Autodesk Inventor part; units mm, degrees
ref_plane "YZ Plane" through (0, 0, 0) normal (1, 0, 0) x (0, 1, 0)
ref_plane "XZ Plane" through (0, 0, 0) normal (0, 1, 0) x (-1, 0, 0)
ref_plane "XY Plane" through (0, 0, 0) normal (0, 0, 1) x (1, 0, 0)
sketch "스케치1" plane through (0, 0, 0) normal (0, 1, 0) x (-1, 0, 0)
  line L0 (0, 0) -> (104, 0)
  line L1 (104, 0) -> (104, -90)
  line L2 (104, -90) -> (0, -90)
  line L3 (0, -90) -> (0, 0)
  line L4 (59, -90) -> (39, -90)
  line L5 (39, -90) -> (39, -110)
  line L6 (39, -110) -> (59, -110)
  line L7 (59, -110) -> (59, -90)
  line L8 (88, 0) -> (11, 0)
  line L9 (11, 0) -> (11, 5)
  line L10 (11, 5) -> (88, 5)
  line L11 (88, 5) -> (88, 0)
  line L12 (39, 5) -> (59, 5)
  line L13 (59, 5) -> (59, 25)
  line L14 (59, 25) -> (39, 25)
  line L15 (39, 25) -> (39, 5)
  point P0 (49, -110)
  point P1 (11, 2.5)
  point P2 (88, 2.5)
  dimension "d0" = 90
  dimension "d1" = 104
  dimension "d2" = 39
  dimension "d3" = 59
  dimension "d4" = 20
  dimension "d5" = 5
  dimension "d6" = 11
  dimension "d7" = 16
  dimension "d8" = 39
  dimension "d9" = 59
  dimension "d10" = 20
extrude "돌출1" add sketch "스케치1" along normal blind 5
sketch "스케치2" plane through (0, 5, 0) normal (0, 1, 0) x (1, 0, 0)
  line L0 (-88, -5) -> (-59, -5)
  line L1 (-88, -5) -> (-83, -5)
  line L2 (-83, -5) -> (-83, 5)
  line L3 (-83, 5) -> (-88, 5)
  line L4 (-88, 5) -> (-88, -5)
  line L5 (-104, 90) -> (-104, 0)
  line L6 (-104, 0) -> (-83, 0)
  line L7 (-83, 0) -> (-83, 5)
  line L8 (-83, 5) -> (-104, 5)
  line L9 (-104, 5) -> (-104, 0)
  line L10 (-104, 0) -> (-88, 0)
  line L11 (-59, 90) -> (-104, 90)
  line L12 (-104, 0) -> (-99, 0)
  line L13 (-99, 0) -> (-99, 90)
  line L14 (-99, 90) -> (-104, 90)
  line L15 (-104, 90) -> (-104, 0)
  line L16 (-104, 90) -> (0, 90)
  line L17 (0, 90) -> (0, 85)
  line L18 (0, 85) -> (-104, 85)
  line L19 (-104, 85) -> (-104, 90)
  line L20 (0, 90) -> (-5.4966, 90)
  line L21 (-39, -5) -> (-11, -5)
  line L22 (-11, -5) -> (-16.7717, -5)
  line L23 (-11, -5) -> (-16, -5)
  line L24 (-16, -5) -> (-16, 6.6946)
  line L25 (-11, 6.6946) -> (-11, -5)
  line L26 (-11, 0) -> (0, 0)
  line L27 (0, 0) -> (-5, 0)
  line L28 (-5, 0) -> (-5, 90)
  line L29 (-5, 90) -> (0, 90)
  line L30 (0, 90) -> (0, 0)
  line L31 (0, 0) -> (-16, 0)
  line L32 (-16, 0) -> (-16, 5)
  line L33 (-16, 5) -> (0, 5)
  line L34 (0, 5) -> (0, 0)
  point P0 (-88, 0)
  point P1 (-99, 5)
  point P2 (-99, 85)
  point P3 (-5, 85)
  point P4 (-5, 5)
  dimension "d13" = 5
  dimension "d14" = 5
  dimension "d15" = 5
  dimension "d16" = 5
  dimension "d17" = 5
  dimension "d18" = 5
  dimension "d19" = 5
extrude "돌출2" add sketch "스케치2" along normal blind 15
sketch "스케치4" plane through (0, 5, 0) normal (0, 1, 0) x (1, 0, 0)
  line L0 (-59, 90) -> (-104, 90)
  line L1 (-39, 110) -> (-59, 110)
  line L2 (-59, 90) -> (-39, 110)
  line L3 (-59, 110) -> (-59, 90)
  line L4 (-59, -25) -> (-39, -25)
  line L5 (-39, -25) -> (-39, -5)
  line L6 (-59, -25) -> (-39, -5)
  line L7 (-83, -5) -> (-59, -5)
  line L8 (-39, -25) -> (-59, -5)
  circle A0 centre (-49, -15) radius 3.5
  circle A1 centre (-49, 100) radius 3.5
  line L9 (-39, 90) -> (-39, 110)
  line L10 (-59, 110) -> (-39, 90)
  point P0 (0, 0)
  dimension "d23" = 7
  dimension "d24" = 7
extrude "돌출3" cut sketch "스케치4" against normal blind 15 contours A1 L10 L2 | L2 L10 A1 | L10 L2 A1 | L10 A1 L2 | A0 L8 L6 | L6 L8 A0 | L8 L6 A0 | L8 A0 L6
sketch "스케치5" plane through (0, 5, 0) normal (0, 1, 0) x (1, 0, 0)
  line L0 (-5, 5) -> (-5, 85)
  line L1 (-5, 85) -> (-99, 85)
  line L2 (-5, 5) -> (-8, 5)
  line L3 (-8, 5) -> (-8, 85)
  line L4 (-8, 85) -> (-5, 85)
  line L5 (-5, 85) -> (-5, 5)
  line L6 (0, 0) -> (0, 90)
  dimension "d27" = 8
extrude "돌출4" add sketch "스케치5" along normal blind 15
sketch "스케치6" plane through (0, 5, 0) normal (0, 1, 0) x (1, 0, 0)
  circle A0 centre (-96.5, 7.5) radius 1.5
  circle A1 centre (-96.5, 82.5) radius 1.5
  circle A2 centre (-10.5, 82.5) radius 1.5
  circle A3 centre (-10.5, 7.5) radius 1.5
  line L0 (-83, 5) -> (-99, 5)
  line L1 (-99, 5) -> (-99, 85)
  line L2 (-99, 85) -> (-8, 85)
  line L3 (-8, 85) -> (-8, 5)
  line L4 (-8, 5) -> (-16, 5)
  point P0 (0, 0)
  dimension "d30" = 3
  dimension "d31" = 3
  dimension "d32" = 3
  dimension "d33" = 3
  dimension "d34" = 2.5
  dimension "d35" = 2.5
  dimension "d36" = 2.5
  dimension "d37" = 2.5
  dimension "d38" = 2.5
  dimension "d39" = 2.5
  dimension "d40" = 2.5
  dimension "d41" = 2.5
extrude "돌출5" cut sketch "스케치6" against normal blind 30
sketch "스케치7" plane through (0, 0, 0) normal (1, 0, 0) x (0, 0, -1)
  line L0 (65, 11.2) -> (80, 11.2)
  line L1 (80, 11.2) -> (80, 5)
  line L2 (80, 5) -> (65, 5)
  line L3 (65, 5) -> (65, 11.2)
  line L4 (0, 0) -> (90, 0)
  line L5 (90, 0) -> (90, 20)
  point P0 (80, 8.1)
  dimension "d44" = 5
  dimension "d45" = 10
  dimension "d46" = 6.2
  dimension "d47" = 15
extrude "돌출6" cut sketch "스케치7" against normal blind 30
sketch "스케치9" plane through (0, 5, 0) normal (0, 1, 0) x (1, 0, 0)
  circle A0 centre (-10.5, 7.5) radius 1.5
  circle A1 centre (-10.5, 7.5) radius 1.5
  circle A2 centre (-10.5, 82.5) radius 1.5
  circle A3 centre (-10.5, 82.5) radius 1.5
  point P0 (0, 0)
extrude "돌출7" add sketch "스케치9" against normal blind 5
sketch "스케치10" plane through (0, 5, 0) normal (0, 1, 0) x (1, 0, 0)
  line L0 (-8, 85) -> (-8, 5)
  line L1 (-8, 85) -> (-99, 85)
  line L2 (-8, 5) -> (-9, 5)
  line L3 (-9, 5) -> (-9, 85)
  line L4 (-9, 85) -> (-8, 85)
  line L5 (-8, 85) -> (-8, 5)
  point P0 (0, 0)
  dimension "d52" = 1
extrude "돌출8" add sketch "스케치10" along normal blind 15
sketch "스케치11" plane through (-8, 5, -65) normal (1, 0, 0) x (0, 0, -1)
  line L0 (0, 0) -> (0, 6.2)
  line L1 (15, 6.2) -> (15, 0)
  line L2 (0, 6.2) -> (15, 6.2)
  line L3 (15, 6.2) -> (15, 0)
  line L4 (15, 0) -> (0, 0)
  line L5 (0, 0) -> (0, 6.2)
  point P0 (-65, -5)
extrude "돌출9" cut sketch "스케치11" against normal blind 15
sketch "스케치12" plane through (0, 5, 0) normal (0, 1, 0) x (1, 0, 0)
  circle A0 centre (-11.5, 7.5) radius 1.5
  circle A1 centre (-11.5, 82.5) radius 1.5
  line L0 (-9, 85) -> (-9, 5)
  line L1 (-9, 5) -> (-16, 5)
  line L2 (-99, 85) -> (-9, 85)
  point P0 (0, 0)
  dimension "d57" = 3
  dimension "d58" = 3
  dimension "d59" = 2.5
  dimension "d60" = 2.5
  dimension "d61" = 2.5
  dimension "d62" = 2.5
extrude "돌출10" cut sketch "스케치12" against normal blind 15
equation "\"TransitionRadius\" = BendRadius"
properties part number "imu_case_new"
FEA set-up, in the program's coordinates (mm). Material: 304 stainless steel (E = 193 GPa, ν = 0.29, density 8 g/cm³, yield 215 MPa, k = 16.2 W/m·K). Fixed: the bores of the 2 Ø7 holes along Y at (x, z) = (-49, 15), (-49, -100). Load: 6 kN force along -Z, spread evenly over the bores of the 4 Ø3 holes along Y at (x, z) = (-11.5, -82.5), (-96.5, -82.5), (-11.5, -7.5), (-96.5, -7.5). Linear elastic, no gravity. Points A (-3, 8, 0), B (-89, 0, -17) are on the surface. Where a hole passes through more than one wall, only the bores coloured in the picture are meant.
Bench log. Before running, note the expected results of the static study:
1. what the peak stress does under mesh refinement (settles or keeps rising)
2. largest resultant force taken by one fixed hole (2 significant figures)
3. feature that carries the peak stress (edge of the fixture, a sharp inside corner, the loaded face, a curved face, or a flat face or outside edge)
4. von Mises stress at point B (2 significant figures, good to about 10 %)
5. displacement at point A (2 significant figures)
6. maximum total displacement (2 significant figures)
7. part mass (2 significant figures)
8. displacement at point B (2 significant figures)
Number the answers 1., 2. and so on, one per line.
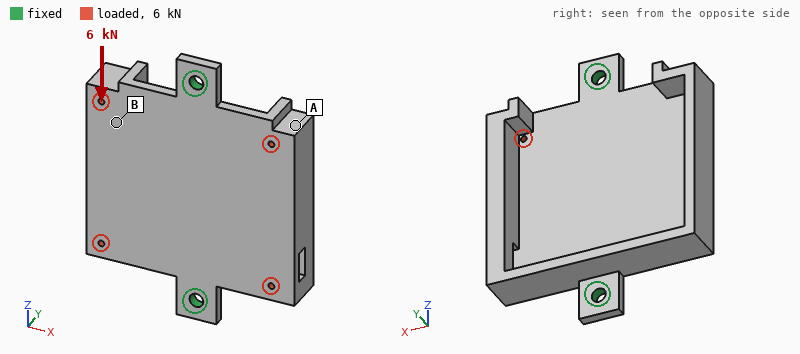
1. keeps rising
2. 3.1 kN
3. edge of the fixture
4. 15 MPa
5. 6.5 µm
6. 12 µm
7. 640 g
8. 7.7 µm
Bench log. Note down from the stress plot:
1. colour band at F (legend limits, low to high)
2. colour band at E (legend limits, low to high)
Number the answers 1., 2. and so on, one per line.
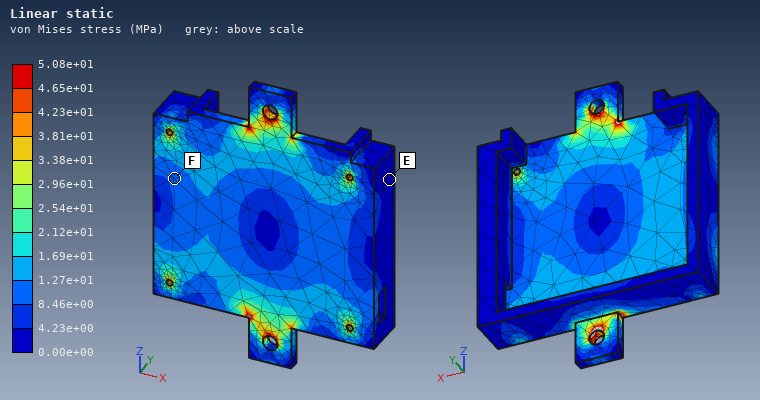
1. 8.46e+00 to 1.27e+01 MPa
2. 0.00e+00 to 4.23e+00 MPa
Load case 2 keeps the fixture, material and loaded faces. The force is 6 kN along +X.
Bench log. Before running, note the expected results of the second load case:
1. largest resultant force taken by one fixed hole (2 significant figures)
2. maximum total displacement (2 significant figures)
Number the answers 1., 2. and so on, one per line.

1. 3.1 kN
2. 13 µm
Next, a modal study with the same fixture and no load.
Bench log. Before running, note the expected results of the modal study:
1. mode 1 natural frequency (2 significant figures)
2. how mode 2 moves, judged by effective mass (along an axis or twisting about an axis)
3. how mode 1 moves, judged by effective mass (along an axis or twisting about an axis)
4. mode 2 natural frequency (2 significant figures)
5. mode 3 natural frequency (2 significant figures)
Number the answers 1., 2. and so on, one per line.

1. 590 Hz
2. along Y
3. twisting about Z
4. 1100 Hz
5. 1800 Hz
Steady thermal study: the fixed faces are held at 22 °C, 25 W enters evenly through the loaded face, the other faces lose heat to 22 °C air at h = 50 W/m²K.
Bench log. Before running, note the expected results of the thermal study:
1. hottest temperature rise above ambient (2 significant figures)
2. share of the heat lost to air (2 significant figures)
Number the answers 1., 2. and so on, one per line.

1. 48 K
2. 93 %
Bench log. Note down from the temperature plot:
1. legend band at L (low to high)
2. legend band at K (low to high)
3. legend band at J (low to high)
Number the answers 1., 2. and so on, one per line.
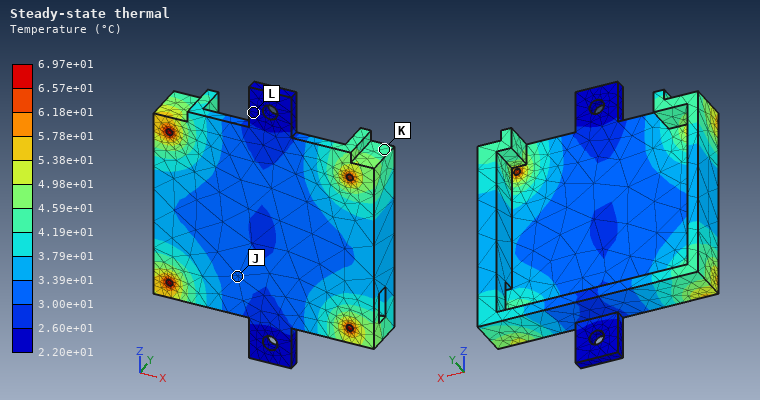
1. 2.20e+01 to 2.60e+01 °C
2. 4.19e+01 to 4.59e+01 °C
3. 3.00e+01 to 3.39e+01 °C
